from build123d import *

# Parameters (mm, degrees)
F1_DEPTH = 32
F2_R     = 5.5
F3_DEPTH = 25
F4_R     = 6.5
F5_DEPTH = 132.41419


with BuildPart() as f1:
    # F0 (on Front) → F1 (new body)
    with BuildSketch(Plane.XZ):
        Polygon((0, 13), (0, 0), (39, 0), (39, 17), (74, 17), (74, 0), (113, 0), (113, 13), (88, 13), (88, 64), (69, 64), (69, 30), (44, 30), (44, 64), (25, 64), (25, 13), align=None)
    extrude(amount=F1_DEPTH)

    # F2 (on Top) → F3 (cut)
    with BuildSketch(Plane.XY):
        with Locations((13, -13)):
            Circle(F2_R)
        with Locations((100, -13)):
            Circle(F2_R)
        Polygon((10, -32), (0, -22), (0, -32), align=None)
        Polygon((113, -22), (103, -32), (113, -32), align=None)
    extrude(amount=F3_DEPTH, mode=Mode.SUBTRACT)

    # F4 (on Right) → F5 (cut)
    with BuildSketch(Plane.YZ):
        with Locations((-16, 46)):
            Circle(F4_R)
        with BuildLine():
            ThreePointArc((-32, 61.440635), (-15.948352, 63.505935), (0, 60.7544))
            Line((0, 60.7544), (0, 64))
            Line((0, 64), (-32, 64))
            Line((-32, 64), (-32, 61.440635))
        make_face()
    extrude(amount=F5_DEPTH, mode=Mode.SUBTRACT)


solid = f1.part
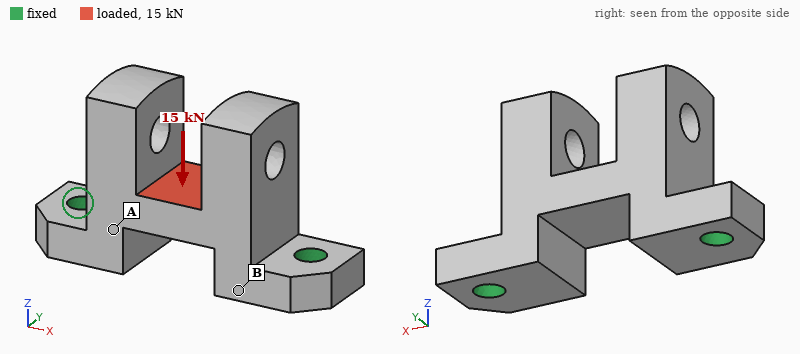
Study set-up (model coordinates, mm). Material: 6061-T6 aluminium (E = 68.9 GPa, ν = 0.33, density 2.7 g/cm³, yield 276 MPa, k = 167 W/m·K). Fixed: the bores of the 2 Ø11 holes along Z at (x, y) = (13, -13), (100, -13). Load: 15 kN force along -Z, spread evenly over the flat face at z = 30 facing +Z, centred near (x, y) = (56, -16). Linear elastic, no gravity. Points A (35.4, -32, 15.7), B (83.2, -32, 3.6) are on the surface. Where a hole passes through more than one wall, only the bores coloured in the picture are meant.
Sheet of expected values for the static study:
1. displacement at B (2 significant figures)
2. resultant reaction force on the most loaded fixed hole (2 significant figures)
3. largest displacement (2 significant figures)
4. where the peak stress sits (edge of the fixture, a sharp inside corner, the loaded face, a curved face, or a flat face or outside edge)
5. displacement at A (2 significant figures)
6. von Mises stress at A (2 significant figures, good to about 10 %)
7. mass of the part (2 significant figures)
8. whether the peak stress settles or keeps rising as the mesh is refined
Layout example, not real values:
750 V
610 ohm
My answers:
29 µm
11 kN
77 µm
edge of the fixture
35 µm
38 MPa
250 g
keeps rising
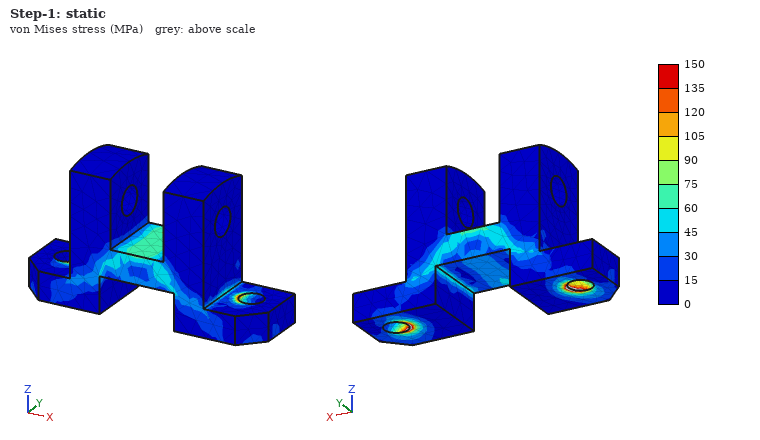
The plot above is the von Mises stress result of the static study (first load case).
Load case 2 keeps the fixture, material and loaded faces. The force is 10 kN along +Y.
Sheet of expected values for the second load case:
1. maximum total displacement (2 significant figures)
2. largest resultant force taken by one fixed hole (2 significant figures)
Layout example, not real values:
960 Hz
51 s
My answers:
0.22 mm
5.0 kN
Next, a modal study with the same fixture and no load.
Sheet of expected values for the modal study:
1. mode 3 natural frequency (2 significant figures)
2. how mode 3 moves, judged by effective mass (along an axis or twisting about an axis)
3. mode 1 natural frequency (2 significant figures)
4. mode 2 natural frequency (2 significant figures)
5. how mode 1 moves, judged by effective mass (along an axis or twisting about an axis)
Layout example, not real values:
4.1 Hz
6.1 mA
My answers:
5700 Hz
along X
2800 Hz
4600 Hz
along Y
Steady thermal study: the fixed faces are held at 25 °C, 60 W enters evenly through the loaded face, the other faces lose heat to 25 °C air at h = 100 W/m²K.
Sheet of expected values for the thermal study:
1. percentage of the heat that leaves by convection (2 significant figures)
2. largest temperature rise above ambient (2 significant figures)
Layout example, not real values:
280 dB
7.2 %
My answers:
23 %
16 K
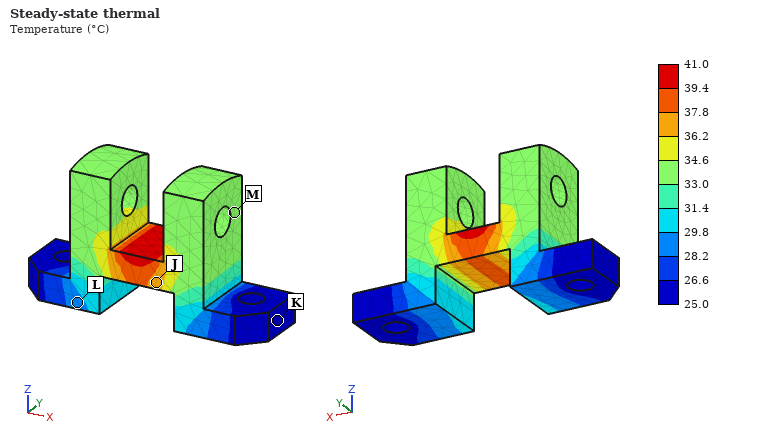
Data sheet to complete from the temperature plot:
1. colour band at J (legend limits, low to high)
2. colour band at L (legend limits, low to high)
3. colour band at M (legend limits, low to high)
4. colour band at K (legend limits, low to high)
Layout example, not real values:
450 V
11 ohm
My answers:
36.2 to 37.8 °C
28.2 to 29.8 °C
33.0 to 34.6 °C
25.0 to 26.6 °C
